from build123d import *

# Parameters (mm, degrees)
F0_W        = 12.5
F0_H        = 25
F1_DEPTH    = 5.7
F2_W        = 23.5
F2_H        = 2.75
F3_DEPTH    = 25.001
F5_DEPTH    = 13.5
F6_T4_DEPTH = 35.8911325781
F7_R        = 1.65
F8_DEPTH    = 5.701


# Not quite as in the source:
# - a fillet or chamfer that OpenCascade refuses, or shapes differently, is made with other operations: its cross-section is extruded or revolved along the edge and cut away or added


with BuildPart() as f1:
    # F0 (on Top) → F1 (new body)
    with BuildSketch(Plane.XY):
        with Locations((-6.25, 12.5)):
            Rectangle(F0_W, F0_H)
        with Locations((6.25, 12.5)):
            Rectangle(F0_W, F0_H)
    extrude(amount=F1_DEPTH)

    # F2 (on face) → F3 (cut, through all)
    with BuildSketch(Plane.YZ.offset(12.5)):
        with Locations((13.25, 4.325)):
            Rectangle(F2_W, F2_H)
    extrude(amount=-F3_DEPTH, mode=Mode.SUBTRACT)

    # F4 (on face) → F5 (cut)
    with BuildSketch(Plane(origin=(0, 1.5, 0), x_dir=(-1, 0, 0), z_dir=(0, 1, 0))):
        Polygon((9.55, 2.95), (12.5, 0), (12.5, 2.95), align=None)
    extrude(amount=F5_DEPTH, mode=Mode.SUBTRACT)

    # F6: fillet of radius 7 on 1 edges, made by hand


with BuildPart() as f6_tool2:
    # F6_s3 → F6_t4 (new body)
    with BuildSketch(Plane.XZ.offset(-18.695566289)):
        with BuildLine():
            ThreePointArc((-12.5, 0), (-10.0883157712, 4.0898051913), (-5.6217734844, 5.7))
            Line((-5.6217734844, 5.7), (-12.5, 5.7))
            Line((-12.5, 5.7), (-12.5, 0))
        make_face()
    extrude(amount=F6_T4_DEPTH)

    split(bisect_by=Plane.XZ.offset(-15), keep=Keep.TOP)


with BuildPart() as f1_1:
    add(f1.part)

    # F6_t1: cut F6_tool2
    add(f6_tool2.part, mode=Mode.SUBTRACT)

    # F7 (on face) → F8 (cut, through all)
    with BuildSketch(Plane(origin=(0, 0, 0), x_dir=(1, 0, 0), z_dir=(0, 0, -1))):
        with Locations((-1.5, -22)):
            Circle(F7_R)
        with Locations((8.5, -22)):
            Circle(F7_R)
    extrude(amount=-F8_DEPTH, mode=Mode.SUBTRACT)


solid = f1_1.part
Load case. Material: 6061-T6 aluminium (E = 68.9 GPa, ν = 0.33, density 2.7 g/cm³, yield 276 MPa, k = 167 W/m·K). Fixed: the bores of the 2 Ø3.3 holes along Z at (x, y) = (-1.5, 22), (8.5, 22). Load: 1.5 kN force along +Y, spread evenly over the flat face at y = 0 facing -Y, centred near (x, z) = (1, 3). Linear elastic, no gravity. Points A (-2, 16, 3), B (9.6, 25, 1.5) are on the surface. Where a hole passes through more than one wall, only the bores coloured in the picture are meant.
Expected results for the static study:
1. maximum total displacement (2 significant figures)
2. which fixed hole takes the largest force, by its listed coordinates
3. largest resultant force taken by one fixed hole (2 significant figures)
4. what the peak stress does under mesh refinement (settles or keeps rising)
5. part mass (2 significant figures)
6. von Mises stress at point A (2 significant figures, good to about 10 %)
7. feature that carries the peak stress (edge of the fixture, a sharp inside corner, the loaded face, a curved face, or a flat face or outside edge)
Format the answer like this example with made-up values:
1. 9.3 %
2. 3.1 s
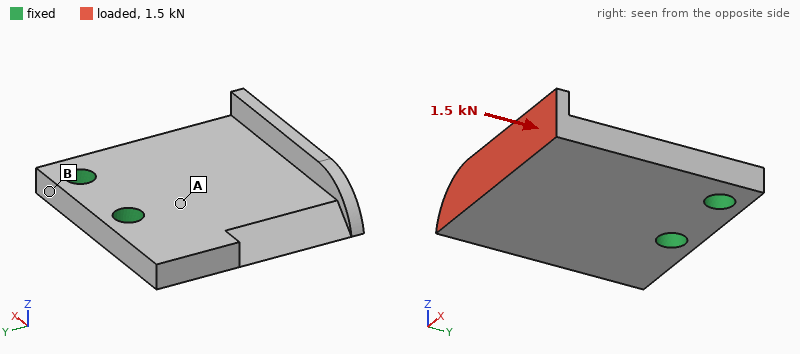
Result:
1. 0.14 mm
2. (-1.5, 22)
3. 1.1 kN
4. keeps rising
5. 4.9 g
6. 88 MPa
7. edge of the fixture
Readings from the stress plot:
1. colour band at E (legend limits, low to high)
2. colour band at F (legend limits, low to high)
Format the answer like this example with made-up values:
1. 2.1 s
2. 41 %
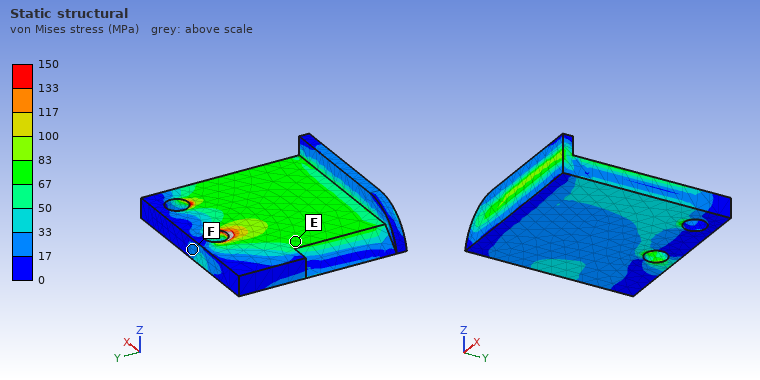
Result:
1. 67 to 83 MPa
2. 17 to 33 MPa
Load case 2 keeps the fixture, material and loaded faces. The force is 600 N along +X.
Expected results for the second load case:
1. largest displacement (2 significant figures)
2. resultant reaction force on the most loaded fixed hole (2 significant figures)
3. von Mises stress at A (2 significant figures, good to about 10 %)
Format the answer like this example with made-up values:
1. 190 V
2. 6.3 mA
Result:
1. 49 µm
2. 1.1 kN
3. 44 MPa
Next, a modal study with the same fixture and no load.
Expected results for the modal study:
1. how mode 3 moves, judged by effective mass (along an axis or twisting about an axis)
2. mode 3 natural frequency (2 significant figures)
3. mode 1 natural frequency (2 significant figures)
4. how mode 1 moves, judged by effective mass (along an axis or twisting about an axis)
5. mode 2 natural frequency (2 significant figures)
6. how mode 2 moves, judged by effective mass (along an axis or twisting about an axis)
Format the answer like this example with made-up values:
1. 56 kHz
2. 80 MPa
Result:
1. along X
2. 17 kHz
3. 4600 Hz
4. along Z
5. 9500 Hz
6. twisting about Y
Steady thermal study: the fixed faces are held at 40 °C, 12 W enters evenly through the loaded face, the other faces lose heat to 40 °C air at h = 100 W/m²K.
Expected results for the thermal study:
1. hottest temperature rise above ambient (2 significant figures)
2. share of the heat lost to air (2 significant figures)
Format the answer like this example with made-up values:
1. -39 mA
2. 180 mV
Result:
1. 22 K
2. 12 %
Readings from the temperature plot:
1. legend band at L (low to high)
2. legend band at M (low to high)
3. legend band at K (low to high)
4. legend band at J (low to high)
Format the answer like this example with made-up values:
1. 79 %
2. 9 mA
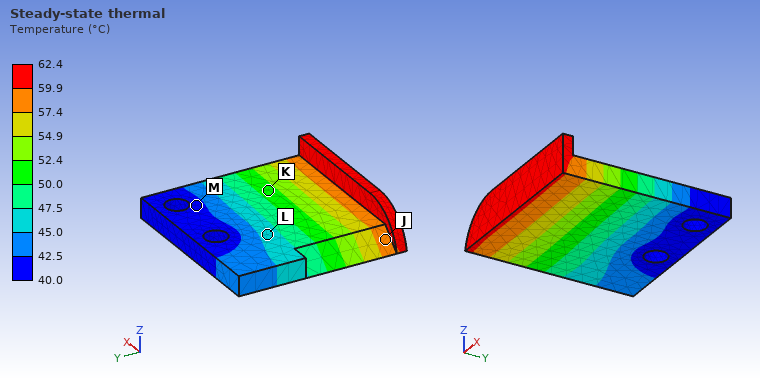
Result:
1. 45.0 to 47.5 °C
2. 40.0 to 42.5 °C
3. 50.0 to 52.4 °C
4. 57.4 to 59.9 °C
